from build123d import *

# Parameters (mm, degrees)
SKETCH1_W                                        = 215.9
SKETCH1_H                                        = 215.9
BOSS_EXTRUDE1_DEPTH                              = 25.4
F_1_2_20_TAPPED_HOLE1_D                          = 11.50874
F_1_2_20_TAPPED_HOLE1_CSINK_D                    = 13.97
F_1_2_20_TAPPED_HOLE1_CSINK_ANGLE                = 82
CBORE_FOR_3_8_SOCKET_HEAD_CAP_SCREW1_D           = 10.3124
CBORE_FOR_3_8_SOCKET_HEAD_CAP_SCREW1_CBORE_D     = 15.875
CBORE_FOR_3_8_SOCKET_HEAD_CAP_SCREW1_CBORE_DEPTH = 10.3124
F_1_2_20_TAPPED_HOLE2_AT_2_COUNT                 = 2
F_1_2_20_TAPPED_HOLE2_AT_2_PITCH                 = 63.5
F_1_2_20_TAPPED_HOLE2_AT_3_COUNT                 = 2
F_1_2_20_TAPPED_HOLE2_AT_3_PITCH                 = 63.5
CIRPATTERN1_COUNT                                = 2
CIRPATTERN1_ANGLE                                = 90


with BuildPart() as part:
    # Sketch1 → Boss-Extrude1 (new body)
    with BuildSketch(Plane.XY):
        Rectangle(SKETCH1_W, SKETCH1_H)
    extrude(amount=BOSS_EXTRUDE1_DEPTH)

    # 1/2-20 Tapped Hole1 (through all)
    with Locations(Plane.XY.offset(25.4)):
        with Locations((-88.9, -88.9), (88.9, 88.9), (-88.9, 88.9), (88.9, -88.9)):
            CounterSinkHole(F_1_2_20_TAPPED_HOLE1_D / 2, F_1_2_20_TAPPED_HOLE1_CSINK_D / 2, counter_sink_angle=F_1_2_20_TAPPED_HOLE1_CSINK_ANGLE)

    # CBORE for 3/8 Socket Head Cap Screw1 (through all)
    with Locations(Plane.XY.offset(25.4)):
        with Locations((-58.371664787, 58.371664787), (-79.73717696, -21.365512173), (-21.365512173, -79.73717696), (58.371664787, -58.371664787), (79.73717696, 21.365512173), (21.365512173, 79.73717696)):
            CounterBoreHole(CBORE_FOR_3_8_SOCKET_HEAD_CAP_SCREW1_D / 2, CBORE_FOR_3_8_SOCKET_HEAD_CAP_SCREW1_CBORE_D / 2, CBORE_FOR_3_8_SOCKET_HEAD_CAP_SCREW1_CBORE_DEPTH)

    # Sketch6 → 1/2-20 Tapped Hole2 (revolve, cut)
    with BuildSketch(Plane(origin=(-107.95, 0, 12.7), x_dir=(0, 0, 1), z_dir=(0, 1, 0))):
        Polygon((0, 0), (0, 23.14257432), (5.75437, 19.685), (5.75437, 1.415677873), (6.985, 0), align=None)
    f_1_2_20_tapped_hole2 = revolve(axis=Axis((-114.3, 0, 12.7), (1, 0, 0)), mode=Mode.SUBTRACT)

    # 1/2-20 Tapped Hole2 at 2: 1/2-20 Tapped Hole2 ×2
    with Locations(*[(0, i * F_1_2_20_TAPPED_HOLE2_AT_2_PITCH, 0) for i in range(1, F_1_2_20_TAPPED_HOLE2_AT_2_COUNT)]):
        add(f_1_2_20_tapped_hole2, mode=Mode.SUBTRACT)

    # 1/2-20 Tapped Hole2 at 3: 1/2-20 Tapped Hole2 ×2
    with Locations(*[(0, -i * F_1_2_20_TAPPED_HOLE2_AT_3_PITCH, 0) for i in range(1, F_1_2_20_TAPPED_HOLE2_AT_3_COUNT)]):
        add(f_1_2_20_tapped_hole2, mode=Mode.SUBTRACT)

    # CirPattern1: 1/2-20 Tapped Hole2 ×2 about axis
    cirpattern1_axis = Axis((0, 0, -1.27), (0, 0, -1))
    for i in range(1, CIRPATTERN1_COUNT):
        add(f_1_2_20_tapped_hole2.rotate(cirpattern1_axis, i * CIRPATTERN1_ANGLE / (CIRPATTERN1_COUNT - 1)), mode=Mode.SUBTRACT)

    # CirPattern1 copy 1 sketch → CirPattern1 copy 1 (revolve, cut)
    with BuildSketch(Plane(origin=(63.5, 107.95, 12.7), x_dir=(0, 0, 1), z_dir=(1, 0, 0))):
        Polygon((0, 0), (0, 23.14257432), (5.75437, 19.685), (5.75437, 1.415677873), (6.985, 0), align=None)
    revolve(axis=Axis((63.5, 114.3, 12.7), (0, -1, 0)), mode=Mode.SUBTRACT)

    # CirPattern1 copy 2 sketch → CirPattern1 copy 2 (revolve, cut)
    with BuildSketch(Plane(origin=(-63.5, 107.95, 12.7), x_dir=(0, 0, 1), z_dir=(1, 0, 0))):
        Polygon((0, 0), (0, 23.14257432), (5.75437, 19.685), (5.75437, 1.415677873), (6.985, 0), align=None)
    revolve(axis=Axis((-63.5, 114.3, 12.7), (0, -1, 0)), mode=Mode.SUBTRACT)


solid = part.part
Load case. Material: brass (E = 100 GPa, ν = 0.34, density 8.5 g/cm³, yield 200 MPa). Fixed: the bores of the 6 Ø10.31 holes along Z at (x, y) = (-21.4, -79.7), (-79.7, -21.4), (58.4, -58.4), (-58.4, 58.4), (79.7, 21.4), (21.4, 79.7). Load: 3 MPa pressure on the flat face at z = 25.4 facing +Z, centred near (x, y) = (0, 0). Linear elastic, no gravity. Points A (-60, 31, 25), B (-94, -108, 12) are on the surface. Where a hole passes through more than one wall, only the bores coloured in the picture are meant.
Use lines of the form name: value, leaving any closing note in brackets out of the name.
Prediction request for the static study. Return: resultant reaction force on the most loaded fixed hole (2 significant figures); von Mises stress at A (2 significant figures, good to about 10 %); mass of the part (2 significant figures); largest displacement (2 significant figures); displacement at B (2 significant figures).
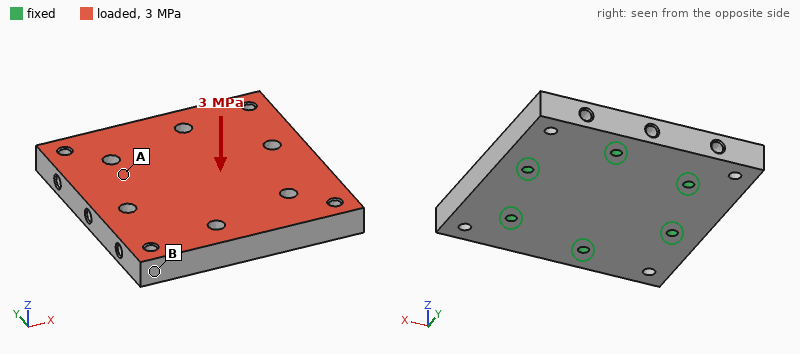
resultant reaction force on the most loaded fixed hole: 24 kN
von Mises stress at A: 20 MPa
mass of the part: 9.7 kg
largest displacement: 81 µm
displacement at B: 69 µm
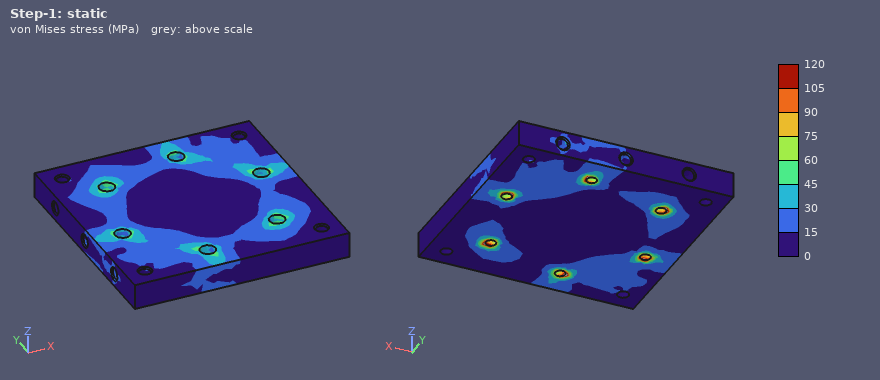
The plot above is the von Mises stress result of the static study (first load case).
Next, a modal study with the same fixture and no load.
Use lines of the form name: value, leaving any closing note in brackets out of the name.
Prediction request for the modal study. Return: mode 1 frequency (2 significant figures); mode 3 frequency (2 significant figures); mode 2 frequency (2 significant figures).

mode 1 frequency: 2600 Hz
mode 3 frequency: 3000 Hz
mode 2 frequency: 2600 Hz
